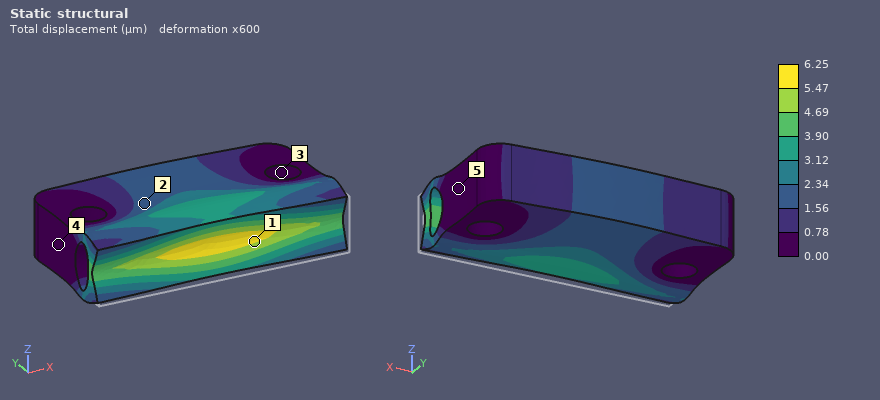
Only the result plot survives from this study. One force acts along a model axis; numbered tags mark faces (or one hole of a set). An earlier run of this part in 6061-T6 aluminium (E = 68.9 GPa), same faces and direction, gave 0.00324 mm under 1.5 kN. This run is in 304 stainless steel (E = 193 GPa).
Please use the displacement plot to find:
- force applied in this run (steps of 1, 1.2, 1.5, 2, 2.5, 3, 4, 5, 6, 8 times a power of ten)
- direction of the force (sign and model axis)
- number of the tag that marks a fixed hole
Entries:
8 kN
+Y
3
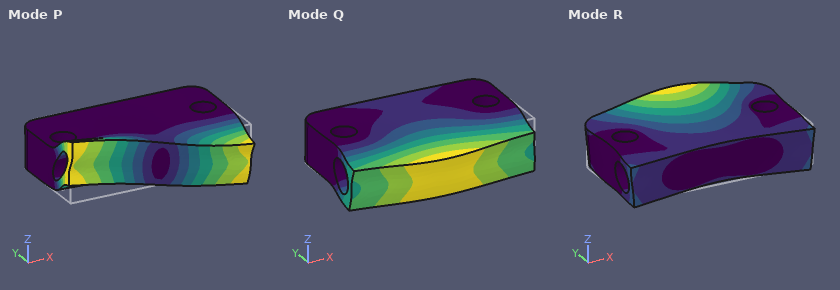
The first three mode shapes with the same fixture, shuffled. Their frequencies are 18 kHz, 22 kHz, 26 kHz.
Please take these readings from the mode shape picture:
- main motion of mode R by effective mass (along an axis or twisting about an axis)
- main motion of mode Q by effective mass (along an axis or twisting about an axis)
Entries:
along Z
along Z
